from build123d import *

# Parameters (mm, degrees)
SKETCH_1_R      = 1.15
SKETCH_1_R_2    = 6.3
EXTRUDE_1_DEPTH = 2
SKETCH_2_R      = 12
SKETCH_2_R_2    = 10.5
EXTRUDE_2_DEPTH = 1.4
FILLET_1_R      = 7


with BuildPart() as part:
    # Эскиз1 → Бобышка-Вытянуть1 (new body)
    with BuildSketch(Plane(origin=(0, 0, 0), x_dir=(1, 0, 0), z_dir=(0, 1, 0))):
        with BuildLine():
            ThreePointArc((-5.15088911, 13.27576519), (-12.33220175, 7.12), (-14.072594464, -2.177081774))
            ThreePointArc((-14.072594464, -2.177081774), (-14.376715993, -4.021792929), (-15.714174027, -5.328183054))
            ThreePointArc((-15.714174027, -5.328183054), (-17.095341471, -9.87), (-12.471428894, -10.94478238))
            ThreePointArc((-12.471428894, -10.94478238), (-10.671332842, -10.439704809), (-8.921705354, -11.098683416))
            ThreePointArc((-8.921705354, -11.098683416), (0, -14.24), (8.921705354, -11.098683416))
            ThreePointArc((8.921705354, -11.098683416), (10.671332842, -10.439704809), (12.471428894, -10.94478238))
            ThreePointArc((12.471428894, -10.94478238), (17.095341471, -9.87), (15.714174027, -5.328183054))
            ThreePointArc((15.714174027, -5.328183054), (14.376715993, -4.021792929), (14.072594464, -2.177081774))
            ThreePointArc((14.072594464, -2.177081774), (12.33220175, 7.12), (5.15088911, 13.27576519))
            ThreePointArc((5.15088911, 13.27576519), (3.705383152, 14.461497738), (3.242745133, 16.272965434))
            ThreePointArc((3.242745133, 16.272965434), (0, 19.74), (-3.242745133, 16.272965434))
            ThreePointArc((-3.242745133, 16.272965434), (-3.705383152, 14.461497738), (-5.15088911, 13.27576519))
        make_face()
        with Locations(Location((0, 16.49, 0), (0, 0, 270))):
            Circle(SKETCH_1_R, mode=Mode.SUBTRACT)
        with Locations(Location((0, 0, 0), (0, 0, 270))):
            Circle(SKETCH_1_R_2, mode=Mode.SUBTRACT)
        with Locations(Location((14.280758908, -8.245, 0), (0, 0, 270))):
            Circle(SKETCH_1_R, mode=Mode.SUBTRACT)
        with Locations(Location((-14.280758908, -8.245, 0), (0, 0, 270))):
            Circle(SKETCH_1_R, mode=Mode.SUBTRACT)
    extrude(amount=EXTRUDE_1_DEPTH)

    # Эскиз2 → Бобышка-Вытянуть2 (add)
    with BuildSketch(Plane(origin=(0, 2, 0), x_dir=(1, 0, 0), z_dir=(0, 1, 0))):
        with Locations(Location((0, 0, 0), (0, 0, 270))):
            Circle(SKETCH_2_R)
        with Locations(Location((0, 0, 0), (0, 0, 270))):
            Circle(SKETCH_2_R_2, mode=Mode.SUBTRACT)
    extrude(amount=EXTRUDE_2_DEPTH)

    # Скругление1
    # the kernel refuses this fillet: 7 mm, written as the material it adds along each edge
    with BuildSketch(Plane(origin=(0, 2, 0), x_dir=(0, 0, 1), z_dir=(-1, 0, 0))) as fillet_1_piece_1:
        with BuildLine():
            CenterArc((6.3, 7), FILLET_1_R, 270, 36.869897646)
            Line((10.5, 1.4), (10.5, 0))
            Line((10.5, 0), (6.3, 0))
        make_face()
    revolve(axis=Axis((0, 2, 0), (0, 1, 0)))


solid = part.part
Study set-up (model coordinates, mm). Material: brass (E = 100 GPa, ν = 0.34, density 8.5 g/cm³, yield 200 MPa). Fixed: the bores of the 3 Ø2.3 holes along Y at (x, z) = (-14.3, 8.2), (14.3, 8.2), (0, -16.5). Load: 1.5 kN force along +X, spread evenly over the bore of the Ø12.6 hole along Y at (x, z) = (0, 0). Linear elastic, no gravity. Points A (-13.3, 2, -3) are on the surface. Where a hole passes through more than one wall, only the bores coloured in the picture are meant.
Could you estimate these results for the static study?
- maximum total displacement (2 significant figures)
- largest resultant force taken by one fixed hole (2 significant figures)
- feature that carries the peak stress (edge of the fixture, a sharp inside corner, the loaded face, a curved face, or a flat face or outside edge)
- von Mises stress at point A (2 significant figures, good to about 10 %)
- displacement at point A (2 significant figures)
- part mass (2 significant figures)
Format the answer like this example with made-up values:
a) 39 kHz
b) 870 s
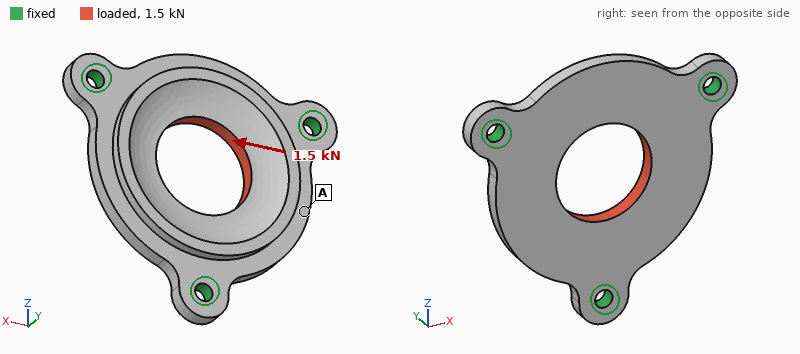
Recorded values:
a) 10 µm
b) 530 N
c) edge of the fixture
d) 24 MPa
e) 7.7 µm
f) 12 g
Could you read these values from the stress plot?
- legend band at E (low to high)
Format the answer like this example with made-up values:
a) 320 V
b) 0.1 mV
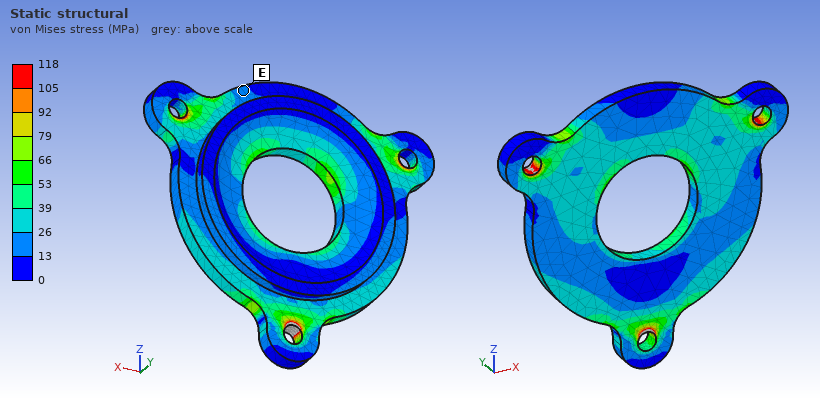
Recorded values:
a) 13 to 26 MPa
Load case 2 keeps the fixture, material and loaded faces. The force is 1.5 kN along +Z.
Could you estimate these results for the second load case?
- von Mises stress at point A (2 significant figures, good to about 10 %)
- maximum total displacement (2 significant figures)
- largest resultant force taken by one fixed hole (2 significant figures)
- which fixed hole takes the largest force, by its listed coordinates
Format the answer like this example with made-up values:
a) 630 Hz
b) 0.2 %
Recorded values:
a) 24 MPa
b) 11 µm
c) 560 N
d) (0, -16.5)
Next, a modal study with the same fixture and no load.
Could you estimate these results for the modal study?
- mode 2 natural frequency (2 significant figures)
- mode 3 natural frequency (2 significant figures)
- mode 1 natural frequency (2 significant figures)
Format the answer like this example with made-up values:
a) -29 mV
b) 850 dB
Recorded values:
a) 9000 Hz
b) 9000 Hz
c) 8900 Hz
